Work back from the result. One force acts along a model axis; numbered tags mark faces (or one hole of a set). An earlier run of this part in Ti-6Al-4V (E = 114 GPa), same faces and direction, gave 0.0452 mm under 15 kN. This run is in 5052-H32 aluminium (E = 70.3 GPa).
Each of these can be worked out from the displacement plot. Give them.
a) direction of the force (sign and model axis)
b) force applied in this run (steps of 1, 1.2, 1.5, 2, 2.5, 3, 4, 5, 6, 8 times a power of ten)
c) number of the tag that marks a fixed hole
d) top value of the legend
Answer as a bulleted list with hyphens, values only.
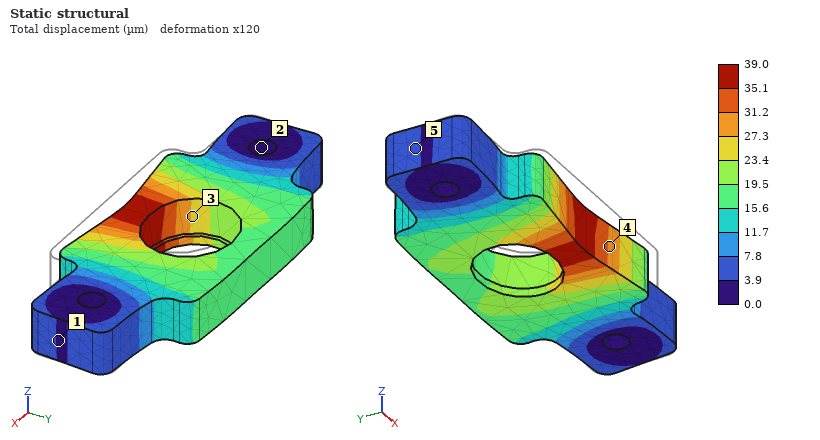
- +Y
- 8 kN
- 2
- 39.0 µm
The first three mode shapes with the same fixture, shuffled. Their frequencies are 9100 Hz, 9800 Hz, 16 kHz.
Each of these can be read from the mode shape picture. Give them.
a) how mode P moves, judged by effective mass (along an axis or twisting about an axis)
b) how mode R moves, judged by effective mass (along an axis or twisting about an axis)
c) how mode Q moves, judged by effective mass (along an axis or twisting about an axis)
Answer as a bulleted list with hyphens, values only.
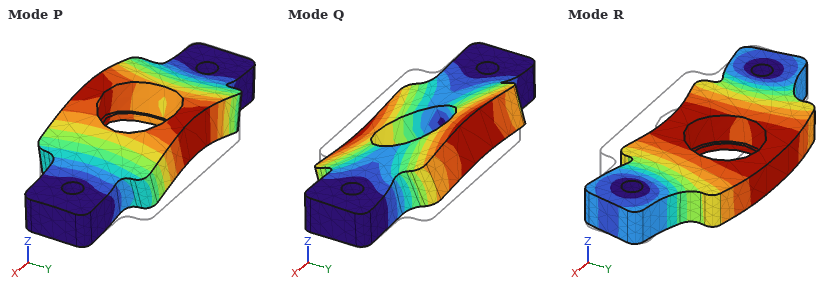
- along Z
- along Y
- twisting about X
